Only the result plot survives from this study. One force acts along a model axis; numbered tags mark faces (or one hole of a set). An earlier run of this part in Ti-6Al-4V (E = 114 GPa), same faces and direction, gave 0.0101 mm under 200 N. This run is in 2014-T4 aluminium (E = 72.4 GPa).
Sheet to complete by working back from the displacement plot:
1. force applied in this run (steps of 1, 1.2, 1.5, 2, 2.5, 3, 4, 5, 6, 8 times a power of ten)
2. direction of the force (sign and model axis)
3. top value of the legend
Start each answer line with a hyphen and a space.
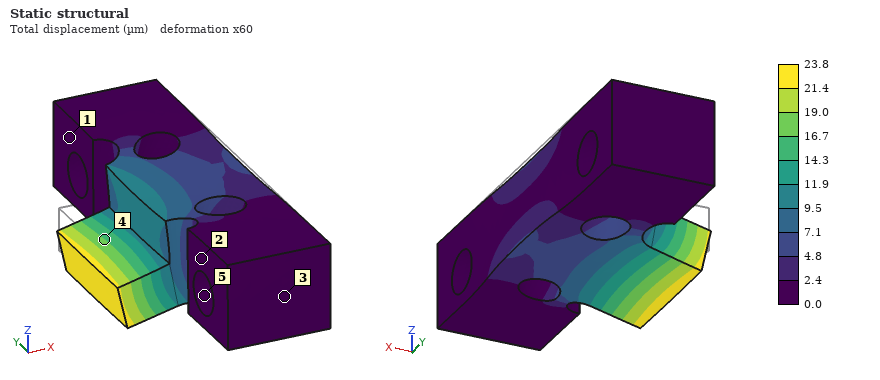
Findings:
- 300 N
- -Z
- 23.8 µm
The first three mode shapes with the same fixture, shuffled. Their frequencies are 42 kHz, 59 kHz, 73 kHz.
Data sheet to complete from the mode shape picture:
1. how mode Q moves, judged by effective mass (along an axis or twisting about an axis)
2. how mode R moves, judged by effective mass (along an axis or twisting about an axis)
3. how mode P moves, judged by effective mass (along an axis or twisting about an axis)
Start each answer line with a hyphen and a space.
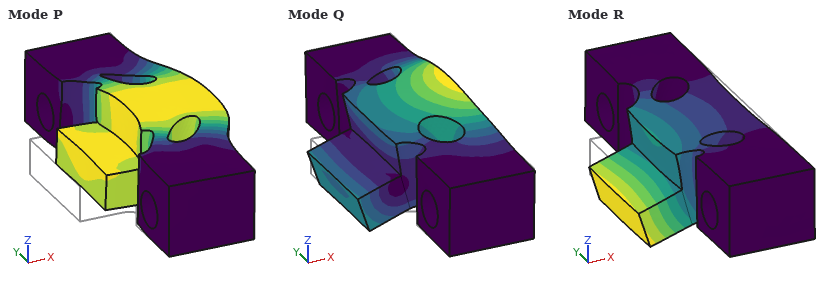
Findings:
- along Z
- along Z
- along X
